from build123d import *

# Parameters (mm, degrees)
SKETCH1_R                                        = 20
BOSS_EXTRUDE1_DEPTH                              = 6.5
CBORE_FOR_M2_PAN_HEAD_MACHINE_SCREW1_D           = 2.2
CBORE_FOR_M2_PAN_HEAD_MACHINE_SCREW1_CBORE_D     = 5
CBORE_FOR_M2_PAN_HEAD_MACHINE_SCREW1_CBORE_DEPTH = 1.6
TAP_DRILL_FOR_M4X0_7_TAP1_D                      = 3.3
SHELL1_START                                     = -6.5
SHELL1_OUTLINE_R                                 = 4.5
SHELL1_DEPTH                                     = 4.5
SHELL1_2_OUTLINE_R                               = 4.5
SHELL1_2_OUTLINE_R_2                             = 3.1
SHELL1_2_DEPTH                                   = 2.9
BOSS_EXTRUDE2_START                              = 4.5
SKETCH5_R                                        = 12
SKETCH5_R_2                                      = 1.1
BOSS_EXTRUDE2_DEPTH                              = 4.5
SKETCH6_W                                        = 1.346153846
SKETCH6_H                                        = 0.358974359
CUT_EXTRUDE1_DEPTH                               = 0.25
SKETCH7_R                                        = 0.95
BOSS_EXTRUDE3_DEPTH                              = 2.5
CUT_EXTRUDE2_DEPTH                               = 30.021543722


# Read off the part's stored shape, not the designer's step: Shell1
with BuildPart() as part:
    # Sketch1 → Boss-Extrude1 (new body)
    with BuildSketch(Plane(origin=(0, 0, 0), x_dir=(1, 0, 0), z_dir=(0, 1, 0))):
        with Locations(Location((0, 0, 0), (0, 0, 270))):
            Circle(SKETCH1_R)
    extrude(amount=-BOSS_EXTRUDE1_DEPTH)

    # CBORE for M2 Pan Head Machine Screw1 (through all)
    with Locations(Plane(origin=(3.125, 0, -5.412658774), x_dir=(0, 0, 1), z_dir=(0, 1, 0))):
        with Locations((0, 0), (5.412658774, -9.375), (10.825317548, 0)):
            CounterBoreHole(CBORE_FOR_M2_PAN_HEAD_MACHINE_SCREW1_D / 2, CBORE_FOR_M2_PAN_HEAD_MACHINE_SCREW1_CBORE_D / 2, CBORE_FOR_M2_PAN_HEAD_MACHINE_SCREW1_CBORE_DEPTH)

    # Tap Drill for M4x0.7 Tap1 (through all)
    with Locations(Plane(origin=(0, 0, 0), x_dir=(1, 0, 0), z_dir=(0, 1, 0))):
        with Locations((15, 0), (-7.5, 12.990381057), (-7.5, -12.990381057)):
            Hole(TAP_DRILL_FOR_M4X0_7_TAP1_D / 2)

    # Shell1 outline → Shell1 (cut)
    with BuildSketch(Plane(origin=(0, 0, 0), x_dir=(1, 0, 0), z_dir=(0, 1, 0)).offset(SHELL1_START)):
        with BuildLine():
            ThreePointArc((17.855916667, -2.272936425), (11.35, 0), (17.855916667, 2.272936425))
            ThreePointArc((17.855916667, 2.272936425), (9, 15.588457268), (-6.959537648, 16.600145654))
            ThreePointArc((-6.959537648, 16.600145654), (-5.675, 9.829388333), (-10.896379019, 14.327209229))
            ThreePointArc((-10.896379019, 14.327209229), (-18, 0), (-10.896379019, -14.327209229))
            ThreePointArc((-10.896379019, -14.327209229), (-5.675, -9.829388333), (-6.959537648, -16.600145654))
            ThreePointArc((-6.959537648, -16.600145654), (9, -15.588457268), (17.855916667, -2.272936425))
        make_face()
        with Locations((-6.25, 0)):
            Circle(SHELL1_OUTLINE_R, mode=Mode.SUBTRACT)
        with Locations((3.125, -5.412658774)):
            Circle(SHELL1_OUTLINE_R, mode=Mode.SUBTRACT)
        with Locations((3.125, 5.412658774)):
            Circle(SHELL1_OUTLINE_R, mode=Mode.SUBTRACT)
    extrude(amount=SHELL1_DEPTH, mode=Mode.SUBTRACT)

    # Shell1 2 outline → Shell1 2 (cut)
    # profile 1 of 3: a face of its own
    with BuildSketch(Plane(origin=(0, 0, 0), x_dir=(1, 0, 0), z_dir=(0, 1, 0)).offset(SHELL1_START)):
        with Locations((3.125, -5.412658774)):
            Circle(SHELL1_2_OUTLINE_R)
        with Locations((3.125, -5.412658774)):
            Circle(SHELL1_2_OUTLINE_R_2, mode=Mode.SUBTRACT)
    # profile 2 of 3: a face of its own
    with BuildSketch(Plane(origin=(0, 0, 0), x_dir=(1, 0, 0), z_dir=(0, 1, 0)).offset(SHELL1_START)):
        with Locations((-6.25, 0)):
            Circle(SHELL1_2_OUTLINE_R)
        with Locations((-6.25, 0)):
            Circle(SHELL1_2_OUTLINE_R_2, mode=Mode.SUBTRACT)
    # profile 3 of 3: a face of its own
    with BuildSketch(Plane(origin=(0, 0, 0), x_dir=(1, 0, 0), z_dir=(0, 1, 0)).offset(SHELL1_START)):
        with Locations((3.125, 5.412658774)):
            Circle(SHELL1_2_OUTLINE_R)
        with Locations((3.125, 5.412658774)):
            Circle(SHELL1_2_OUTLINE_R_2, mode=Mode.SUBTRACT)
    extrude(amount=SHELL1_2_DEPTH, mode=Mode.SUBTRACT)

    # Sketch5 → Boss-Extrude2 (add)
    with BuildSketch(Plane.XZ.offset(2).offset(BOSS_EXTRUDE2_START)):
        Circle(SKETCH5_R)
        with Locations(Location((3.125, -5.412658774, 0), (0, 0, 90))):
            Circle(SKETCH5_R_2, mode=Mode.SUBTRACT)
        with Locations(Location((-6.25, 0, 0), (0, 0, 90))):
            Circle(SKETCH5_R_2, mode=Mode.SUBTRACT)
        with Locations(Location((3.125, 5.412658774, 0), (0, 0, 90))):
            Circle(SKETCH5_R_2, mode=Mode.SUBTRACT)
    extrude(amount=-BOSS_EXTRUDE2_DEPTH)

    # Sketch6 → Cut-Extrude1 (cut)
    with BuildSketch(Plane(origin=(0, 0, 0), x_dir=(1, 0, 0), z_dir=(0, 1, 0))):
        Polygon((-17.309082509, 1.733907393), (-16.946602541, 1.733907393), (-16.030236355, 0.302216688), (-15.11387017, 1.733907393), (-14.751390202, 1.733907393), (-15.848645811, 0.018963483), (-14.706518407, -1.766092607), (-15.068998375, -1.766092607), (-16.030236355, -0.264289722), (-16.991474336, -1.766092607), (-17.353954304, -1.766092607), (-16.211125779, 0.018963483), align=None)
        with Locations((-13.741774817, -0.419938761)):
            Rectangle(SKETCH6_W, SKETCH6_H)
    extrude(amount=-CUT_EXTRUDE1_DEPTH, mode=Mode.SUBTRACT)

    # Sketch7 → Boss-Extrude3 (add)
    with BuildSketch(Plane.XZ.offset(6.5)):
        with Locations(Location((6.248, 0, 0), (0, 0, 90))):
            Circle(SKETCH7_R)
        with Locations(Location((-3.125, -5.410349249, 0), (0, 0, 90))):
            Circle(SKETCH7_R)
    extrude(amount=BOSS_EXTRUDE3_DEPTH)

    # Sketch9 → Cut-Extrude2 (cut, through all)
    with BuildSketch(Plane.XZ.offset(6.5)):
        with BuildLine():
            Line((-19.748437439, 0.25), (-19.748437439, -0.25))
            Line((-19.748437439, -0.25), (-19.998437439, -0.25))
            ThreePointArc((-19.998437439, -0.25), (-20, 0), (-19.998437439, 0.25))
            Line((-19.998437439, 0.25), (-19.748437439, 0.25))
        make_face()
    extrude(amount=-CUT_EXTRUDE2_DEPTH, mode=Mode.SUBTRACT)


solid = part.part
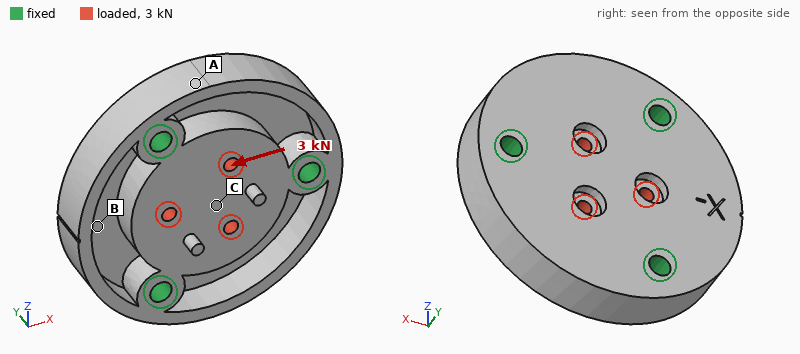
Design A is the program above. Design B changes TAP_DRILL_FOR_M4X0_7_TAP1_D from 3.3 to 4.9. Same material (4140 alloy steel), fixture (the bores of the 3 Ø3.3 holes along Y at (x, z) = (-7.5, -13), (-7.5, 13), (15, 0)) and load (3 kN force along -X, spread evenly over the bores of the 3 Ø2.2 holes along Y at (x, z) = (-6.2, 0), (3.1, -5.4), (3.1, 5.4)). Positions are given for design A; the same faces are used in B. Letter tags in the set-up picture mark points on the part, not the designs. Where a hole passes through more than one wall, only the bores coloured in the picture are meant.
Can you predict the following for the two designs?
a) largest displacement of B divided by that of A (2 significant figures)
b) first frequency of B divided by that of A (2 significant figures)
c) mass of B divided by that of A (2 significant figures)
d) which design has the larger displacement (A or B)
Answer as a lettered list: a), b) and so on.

a) 0.90
b) 1.1
c) 0.97
d) A
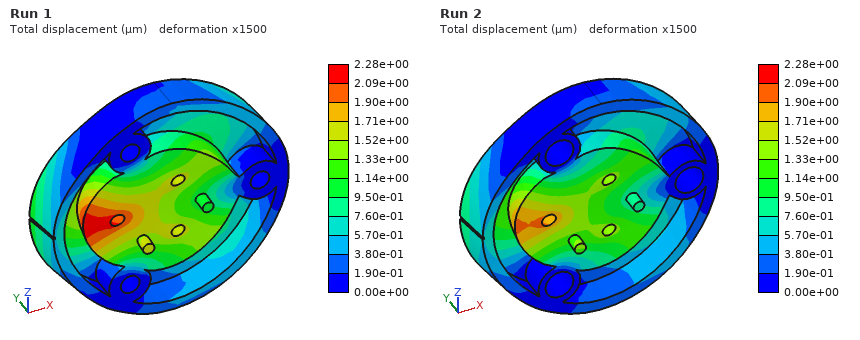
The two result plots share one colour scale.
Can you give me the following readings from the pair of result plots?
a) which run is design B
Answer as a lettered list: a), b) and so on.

a) Run 2
